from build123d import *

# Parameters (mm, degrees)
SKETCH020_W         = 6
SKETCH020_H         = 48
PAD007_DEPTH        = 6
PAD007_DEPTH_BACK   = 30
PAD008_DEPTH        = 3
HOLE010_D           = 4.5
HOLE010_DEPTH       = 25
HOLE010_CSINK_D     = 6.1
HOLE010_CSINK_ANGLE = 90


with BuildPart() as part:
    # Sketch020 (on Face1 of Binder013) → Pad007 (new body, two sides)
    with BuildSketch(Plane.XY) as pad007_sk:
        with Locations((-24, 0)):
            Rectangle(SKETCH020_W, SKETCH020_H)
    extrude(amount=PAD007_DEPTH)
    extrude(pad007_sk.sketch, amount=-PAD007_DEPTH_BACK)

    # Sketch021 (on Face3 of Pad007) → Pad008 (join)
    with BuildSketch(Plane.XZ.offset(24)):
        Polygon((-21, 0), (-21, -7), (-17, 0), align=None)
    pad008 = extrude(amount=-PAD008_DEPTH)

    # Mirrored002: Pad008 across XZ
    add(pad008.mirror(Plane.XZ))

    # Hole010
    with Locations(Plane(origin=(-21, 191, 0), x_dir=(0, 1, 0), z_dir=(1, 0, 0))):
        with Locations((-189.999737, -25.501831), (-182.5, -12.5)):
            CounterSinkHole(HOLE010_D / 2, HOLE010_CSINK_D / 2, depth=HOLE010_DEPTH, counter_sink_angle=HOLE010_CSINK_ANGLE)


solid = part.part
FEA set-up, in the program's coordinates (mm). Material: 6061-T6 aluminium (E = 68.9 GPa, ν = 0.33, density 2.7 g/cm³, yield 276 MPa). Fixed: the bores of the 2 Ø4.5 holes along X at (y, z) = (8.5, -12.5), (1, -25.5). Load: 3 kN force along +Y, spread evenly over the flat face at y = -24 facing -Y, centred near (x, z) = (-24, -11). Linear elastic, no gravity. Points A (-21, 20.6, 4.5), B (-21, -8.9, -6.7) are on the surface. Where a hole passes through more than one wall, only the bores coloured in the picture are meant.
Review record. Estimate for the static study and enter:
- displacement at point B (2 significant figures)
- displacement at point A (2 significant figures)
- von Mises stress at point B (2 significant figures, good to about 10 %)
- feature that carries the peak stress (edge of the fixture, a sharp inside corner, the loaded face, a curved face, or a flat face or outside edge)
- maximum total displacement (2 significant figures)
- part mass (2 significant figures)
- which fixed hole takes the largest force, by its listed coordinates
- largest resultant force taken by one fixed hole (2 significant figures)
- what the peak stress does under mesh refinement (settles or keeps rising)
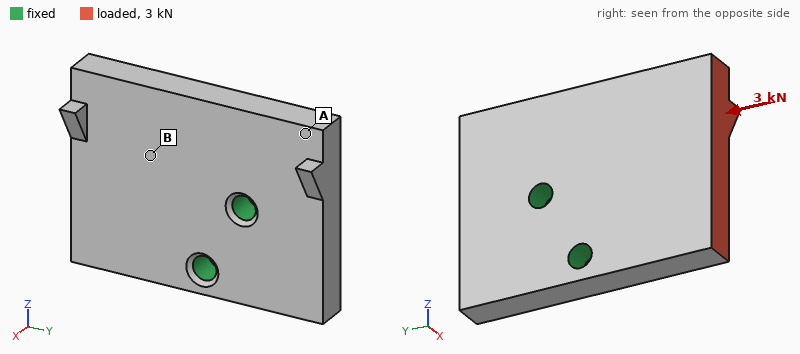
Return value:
11 µm
11 µm
21 MPa
edge of the fixture
30 µm
28 g
(8.5, -12.5)
2.7 kN
keeps rising
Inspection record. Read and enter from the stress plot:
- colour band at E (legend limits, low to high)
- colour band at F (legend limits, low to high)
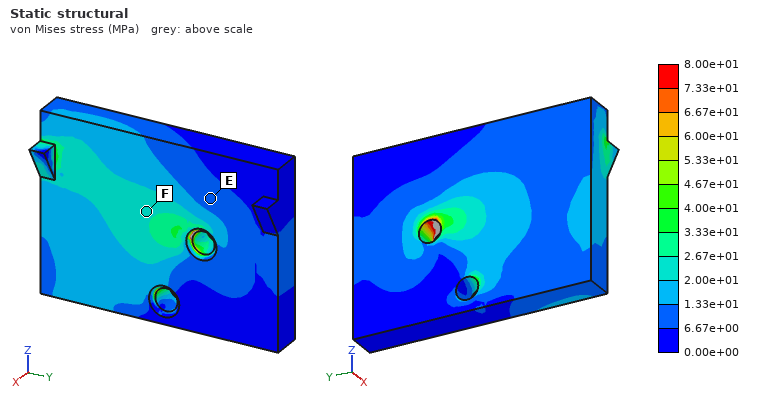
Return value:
6.67e+00 to 1.33e+01 MPa
2.00e+01 to 2.67e+01 MPa
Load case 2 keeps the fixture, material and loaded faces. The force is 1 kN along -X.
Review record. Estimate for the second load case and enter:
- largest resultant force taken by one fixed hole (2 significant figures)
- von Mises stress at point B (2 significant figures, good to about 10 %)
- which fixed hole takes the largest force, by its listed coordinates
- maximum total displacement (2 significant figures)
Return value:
850 N
57 MPa
(1, -25.5)
0.26 mm
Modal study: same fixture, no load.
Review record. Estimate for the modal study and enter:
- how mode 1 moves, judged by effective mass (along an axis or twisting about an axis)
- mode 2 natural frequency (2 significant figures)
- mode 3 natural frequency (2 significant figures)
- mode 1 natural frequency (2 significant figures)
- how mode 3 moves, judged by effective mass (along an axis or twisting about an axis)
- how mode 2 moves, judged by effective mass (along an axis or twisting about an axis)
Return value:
along X
9800 Hz
12 kHz
4900 Hz
along X
twisting about Y
